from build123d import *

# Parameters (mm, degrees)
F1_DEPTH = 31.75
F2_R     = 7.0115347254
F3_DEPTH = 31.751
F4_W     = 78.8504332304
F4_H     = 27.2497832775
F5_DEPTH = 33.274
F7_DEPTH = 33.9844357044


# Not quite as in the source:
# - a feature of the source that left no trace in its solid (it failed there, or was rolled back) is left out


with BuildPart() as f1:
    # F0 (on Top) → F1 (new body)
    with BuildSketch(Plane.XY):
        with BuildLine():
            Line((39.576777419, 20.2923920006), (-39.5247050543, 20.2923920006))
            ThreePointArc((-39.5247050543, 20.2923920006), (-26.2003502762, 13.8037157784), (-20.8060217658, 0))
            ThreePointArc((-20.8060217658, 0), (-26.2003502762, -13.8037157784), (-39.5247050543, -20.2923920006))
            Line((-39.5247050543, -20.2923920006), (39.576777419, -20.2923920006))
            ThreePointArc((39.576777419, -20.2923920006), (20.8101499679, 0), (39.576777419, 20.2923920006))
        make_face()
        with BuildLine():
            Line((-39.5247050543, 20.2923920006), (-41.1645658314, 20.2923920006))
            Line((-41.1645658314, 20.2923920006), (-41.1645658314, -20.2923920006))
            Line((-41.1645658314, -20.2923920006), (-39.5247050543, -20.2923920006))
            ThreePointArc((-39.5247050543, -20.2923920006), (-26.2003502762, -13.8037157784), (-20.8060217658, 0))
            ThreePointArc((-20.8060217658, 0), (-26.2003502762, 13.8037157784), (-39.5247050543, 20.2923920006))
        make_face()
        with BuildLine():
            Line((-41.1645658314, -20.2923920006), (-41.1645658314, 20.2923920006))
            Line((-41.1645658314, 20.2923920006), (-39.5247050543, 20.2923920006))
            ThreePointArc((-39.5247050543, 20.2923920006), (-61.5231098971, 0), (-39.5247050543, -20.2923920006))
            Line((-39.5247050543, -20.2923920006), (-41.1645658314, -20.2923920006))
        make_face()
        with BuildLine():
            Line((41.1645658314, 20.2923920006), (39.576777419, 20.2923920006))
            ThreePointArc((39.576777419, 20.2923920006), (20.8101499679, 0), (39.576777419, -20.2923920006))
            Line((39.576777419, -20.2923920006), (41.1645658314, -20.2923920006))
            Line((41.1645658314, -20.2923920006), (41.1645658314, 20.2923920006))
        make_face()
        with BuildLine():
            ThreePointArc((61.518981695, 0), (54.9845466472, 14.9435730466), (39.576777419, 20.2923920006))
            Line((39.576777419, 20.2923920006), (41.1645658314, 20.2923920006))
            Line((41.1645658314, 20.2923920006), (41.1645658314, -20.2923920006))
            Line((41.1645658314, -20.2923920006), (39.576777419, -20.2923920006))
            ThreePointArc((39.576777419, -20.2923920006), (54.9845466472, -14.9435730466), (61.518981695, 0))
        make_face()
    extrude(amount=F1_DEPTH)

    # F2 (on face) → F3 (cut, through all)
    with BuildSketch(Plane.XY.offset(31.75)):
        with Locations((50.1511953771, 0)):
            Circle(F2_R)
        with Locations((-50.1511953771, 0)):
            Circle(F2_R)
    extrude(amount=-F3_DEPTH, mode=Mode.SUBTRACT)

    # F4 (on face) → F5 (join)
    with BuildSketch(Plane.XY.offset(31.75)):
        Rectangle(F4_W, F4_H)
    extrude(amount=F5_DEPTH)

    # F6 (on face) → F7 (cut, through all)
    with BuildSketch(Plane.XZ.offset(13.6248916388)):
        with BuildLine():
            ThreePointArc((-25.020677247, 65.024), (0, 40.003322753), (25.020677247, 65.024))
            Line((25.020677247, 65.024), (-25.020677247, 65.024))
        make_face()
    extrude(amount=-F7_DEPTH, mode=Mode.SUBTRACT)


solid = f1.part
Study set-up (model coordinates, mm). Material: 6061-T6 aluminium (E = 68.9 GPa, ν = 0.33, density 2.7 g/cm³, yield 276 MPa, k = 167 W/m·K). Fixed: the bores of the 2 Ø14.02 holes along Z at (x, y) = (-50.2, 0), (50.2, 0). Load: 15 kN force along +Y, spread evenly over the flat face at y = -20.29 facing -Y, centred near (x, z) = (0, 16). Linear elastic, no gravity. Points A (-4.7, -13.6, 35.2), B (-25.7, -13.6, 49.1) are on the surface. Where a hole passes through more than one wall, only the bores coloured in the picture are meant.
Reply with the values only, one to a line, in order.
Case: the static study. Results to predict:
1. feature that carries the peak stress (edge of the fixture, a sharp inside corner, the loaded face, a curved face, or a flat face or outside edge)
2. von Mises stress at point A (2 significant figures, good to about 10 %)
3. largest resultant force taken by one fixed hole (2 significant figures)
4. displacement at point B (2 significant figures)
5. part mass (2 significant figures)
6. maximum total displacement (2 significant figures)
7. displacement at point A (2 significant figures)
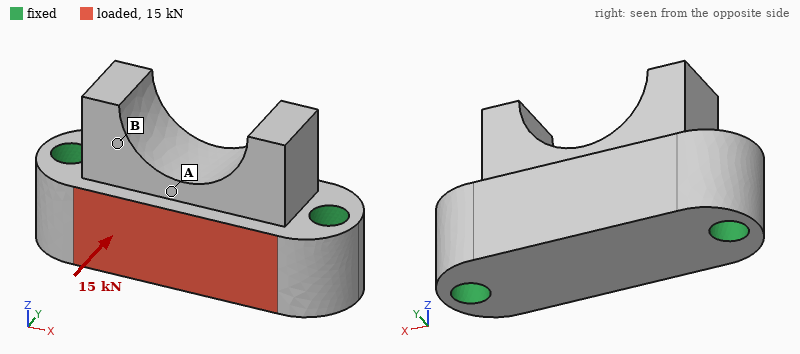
edge of the fixture
8.9 MPa
7.6 kN
8.8 µm
490 g
15 µm
12 µm
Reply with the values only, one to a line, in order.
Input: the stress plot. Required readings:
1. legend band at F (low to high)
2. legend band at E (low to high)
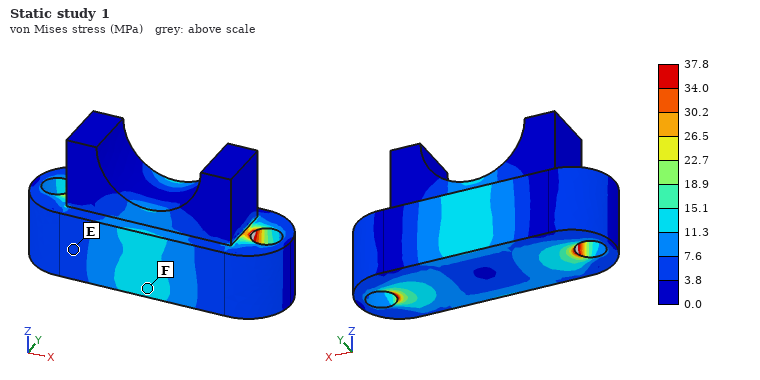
11.3 to 15.1 MPa
3.8 to 7.6 MPa
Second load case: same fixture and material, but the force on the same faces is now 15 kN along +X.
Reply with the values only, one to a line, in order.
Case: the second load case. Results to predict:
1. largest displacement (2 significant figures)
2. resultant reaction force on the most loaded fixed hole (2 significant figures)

5.7 µm
8.0 kN
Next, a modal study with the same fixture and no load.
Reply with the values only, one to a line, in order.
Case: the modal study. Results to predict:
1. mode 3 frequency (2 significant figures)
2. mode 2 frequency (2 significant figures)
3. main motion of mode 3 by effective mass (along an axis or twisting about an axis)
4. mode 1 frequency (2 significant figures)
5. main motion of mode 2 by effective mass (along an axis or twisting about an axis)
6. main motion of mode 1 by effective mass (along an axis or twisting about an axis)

11 kHz
10 kHz
along Y
7800 Hz
along Z
along Y
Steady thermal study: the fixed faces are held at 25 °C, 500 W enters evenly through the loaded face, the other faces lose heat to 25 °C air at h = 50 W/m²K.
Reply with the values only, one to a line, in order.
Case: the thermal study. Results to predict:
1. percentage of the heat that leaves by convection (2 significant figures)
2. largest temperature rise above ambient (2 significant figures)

3.3 %
45 K
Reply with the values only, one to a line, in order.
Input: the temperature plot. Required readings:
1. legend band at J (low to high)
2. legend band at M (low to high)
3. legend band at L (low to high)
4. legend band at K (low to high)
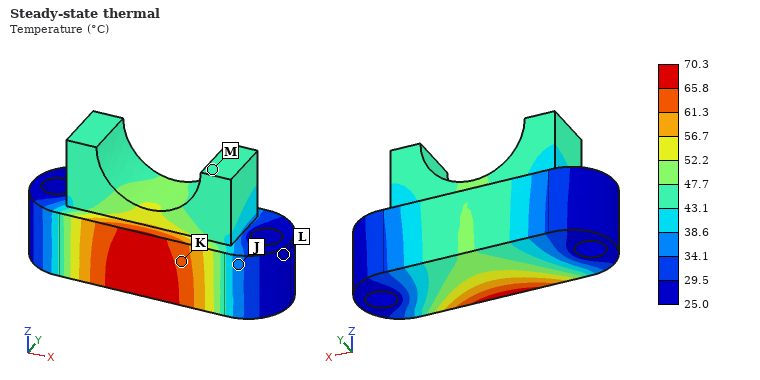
34.1 to 38.6 °C
43.1 to 47.7 °C
25.0 to 29.5 °C
61.3 to 65.8 °C
